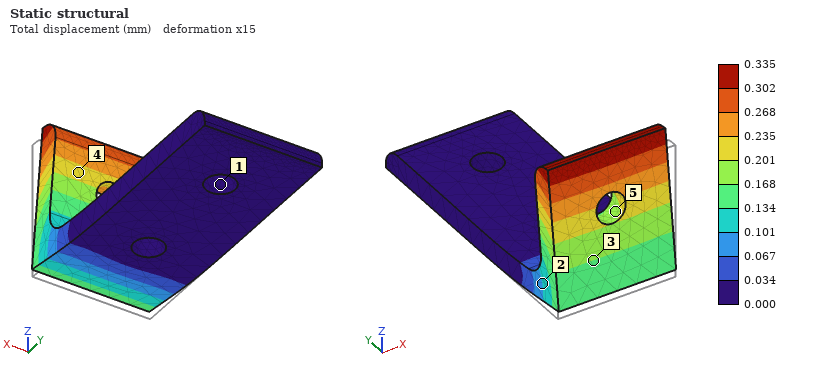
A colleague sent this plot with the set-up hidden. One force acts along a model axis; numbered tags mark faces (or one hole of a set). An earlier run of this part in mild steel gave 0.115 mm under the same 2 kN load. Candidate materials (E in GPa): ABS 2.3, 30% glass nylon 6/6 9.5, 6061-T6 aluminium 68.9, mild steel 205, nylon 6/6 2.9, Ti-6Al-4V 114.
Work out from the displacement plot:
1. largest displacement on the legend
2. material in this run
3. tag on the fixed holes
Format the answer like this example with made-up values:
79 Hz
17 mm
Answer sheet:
0.335 mm
6061-T6 aluminium
1
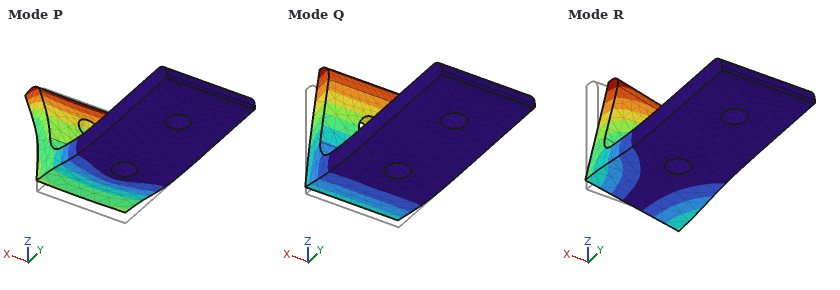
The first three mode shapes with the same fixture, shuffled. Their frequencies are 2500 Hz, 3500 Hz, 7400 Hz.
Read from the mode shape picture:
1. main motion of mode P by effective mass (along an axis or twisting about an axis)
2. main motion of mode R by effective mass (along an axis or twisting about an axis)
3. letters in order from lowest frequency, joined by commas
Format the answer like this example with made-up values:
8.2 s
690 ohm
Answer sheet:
along Z
along X
Q, R, P
